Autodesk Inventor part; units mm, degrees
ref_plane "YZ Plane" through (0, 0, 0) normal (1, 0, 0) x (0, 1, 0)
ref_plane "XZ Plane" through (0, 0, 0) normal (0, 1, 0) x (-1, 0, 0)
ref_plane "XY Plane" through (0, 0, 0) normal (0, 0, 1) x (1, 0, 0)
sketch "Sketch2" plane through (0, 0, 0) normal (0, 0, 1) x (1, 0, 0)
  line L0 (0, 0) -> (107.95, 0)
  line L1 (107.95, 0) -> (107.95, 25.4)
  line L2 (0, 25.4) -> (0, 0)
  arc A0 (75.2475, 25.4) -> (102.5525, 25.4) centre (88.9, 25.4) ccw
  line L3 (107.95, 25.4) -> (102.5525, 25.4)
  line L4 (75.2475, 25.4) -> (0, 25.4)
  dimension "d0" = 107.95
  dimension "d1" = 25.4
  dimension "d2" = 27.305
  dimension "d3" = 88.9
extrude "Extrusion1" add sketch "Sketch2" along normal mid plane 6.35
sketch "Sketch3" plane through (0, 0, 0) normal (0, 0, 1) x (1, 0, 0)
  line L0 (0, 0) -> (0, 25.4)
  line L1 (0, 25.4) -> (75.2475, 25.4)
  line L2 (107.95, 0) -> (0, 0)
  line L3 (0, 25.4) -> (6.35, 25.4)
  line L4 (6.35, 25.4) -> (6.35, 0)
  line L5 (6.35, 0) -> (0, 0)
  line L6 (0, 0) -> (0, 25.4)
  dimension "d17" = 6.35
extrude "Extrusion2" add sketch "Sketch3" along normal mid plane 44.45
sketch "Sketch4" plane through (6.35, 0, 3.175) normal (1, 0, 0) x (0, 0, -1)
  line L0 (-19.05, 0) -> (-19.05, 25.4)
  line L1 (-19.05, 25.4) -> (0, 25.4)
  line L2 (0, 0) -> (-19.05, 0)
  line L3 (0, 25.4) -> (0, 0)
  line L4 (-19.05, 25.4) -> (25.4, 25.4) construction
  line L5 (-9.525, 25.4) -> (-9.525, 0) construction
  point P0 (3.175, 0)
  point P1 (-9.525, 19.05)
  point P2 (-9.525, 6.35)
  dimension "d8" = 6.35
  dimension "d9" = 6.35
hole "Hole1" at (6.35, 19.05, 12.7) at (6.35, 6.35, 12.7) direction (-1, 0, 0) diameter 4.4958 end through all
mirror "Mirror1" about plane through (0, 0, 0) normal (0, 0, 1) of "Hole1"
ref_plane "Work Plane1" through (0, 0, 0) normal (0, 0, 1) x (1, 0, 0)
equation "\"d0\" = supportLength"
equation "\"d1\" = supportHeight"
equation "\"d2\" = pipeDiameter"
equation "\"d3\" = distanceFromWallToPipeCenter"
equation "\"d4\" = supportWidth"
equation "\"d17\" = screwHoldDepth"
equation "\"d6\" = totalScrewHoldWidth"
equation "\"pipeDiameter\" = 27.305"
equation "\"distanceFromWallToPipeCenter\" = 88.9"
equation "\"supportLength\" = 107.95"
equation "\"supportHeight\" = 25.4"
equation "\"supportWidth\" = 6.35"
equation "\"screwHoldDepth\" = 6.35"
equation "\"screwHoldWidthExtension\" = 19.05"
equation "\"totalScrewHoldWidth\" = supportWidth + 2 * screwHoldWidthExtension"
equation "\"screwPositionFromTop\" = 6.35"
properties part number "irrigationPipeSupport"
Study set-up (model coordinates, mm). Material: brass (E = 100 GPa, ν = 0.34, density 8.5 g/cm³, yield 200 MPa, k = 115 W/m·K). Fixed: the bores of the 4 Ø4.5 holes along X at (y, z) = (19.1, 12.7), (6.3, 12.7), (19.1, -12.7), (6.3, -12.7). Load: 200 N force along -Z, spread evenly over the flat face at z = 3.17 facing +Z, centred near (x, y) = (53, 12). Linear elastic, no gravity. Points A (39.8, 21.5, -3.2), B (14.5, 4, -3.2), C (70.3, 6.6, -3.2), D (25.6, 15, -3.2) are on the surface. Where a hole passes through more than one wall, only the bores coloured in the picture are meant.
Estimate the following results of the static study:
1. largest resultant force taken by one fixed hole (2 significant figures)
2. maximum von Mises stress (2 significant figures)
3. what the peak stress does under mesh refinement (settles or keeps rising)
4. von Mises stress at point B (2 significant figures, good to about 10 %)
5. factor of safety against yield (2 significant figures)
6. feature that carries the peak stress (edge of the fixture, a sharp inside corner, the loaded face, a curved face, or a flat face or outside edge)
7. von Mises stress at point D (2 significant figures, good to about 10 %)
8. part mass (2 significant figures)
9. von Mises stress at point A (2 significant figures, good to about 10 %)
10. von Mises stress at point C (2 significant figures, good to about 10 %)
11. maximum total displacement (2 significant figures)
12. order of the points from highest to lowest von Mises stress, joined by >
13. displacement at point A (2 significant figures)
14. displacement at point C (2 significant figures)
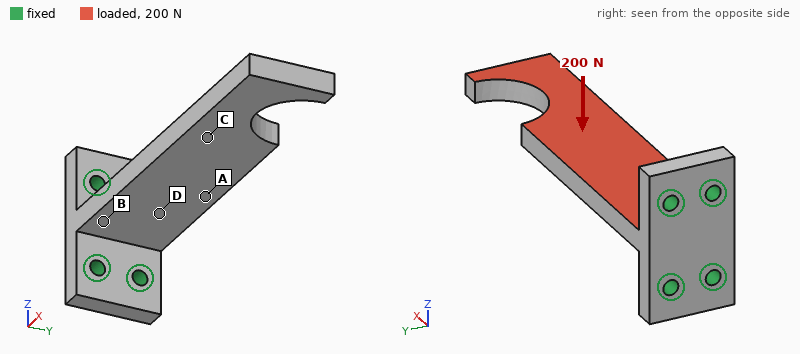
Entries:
290 N
49 MPa
settles
45 MPa
4.1
a flat face or outside edge
34 MPa
180 g
23 MPa
8.1 MPa
0.48 mm
B > D > A > C
0.091 mm
0.25 mm
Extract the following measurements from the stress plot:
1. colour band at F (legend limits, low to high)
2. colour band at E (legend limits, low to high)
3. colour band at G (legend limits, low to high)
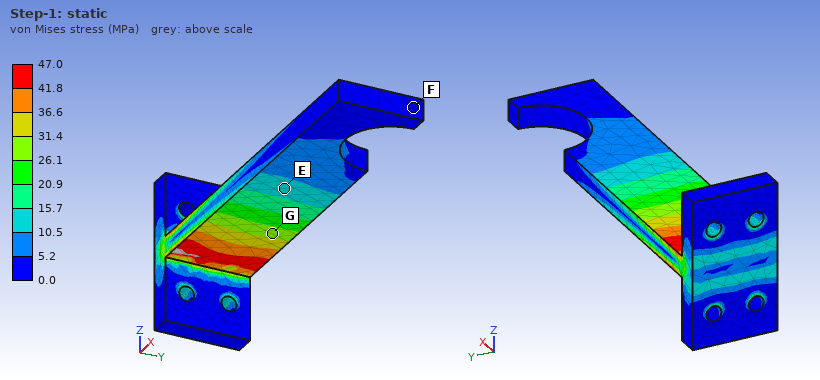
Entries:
0.0 to 5.2 MPa
10.5 to 15.7 MPa
26.1 to 31.4 MPa
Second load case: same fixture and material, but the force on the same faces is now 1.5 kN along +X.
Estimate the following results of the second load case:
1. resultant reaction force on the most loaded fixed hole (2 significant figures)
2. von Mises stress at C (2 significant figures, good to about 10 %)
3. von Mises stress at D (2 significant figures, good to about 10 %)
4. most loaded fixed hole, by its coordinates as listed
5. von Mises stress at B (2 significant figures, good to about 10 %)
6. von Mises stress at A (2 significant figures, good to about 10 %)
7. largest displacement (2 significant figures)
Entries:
550 N
6.3 MPa
14 MPa
(6.3, 12.7)
16 MPa
13 MPa
0.32 mm
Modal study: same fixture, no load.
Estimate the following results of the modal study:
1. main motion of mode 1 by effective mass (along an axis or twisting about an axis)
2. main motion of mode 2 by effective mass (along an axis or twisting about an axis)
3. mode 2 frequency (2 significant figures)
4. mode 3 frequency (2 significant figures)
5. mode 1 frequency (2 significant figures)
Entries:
along Z
along Y
1000 Hz
1900 Hz
370 Hz
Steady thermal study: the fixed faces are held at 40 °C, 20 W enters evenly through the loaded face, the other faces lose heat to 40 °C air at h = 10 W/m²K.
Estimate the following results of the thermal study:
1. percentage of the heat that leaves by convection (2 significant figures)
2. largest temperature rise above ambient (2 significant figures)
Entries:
7.6 %
56 K
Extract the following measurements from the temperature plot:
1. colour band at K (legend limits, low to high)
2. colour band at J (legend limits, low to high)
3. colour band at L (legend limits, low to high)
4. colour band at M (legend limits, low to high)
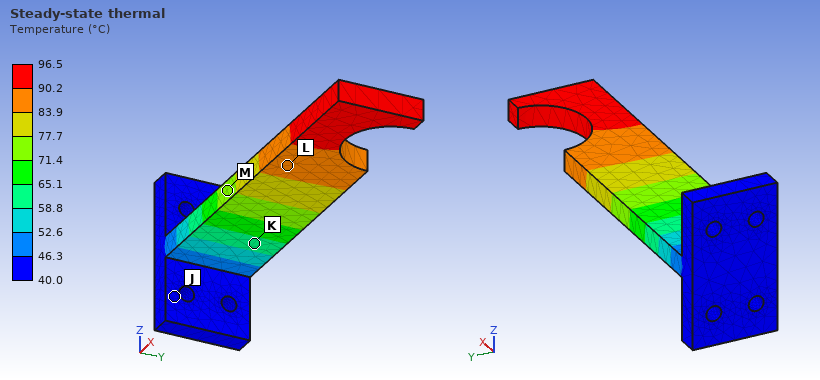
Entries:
58.8 to 65.1 °C
40.0 to 46.3 °C
83.9 to 90.2 °C
71.4 to 77.7 °C
